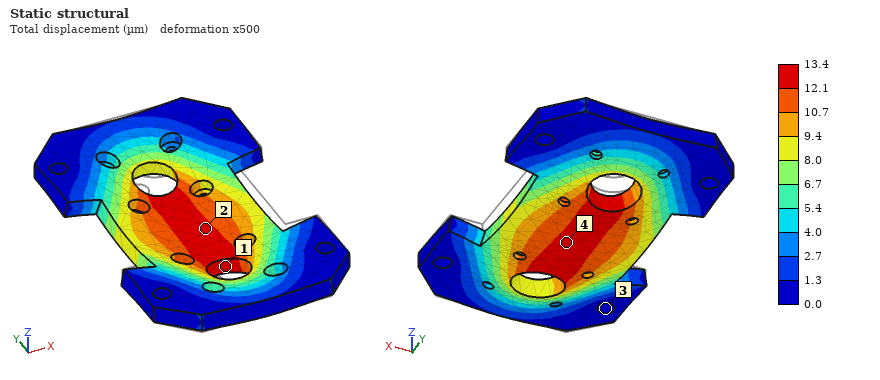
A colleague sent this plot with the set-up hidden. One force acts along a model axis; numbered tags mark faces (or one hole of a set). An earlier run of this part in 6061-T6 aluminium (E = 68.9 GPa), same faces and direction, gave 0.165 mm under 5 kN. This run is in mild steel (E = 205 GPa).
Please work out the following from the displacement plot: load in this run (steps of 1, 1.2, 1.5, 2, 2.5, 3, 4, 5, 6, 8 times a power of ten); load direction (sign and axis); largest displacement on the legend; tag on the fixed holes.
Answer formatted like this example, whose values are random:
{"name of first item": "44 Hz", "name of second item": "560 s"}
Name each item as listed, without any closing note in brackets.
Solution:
{"load in this run": "1.2 kN", "load direction": "-Z", "largest displacement on the legend": "13.4 µm", "tag on the fixed holes": "3"}
